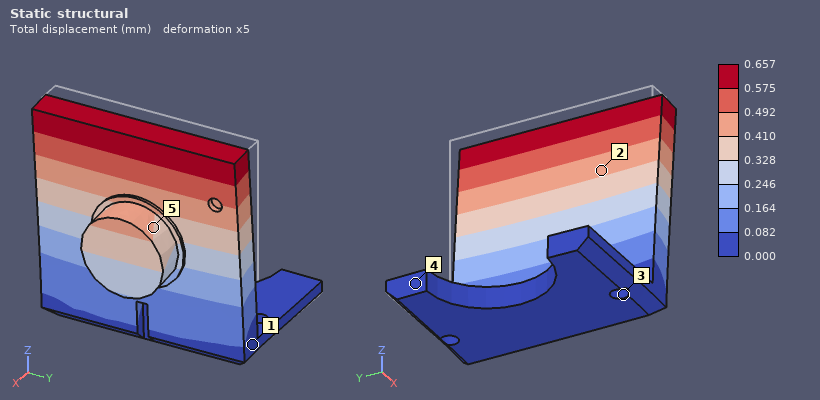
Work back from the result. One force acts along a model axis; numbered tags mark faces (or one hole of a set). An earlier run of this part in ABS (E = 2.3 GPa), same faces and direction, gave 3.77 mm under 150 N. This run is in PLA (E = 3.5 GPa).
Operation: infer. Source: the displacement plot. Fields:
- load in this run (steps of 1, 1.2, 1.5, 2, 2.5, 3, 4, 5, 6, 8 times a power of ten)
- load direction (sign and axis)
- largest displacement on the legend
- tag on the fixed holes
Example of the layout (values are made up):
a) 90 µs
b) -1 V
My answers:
a) 40 N
b) +X
c) 0.657 mm
d) 3
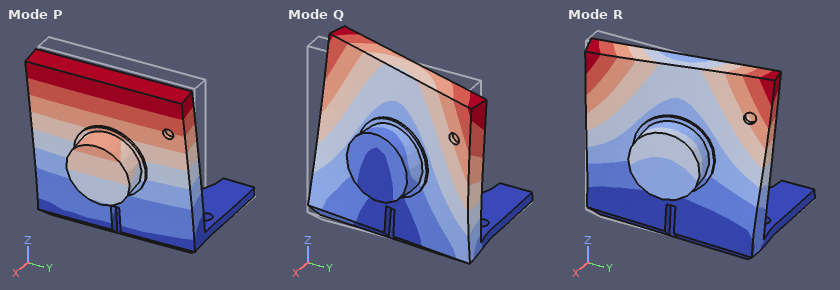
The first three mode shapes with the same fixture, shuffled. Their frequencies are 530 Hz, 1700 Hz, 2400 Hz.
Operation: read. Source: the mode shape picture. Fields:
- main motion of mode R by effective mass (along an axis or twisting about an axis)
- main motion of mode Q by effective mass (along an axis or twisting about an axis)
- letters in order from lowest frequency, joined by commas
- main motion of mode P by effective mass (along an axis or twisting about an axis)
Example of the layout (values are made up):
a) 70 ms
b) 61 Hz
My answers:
a) along Y
b) along Y
c) P, Q, R
d) along X
